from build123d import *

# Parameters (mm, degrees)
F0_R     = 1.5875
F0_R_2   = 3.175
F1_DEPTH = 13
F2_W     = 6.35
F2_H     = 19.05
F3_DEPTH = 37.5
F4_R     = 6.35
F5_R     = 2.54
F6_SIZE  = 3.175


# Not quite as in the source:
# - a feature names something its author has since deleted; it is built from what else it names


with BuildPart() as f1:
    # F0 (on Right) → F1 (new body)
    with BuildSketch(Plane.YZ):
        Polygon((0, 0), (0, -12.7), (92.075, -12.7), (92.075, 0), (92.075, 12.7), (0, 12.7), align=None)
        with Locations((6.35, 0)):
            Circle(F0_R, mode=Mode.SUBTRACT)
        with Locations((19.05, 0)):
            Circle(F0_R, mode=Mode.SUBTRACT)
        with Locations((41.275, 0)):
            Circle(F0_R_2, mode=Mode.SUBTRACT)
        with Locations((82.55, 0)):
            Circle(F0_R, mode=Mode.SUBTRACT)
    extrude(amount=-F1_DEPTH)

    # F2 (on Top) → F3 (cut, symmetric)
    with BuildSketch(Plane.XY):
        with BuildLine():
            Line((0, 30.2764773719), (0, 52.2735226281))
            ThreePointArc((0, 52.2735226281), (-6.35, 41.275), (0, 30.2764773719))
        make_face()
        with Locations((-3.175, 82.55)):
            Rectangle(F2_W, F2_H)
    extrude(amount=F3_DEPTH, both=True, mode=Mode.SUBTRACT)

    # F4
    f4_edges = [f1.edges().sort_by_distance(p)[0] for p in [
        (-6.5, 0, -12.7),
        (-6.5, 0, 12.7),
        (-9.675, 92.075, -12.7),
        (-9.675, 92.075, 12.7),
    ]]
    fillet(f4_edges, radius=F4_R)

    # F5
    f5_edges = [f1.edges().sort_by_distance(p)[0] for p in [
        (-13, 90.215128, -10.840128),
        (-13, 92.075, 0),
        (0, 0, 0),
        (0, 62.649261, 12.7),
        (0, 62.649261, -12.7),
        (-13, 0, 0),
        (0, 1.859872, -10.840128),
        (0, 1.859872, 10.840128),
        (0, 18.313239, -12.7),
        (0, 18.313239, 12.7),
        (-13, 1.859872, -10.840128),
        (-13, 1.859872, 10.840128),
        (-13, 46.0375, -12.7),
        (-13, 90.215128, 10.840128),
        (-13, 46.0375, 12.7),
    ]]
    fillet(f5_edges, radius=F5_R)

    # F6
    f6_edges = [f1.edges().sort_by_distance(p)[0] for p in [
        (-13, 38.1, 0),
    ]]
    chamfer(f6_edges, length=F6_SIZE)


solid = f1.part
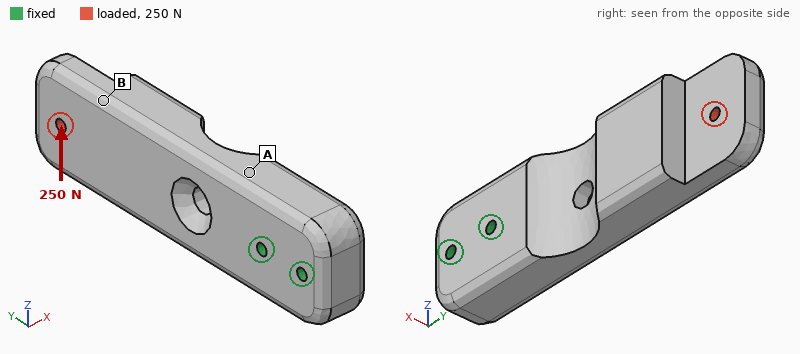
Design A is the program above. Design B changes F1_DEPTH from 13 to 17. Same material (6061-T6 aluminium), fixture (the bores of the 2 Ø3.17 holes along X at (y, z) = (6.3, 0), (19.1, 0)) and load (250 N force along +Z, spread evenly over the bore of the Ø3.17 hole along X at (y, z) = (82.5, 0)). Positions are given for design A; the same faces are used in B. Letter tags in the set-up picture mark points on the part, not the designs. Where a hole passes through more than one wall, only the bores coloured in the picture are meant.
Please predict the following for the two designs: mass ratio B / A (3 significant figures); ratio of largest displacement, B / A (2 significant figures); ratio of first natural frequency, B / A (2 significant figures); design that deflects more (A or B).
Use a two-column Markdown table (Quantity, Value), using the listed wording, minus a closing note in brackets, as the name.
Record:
| Quantity | Value |
|---|---|
| mass ratio B / A | 1.38 |
| ratio of largest displacement, B / A | 0.70 |
| ratio of first natural frequency, B / A | 1.4 |
| design that deflects more | A |
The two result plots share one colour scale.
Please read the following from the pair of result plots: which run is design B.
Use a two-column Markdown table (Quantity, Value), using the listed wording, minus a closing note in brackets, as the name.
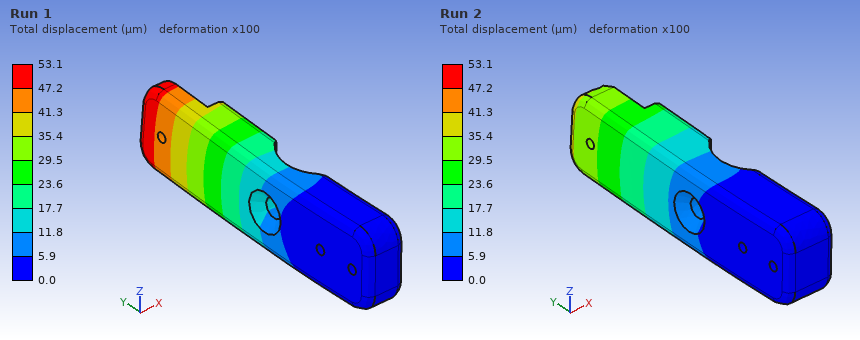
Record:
| Quantity | Value |
|---|---|
| which run is design B | Run 2 |
